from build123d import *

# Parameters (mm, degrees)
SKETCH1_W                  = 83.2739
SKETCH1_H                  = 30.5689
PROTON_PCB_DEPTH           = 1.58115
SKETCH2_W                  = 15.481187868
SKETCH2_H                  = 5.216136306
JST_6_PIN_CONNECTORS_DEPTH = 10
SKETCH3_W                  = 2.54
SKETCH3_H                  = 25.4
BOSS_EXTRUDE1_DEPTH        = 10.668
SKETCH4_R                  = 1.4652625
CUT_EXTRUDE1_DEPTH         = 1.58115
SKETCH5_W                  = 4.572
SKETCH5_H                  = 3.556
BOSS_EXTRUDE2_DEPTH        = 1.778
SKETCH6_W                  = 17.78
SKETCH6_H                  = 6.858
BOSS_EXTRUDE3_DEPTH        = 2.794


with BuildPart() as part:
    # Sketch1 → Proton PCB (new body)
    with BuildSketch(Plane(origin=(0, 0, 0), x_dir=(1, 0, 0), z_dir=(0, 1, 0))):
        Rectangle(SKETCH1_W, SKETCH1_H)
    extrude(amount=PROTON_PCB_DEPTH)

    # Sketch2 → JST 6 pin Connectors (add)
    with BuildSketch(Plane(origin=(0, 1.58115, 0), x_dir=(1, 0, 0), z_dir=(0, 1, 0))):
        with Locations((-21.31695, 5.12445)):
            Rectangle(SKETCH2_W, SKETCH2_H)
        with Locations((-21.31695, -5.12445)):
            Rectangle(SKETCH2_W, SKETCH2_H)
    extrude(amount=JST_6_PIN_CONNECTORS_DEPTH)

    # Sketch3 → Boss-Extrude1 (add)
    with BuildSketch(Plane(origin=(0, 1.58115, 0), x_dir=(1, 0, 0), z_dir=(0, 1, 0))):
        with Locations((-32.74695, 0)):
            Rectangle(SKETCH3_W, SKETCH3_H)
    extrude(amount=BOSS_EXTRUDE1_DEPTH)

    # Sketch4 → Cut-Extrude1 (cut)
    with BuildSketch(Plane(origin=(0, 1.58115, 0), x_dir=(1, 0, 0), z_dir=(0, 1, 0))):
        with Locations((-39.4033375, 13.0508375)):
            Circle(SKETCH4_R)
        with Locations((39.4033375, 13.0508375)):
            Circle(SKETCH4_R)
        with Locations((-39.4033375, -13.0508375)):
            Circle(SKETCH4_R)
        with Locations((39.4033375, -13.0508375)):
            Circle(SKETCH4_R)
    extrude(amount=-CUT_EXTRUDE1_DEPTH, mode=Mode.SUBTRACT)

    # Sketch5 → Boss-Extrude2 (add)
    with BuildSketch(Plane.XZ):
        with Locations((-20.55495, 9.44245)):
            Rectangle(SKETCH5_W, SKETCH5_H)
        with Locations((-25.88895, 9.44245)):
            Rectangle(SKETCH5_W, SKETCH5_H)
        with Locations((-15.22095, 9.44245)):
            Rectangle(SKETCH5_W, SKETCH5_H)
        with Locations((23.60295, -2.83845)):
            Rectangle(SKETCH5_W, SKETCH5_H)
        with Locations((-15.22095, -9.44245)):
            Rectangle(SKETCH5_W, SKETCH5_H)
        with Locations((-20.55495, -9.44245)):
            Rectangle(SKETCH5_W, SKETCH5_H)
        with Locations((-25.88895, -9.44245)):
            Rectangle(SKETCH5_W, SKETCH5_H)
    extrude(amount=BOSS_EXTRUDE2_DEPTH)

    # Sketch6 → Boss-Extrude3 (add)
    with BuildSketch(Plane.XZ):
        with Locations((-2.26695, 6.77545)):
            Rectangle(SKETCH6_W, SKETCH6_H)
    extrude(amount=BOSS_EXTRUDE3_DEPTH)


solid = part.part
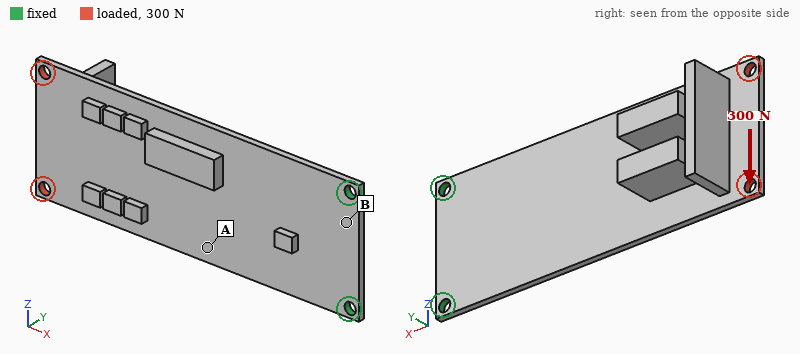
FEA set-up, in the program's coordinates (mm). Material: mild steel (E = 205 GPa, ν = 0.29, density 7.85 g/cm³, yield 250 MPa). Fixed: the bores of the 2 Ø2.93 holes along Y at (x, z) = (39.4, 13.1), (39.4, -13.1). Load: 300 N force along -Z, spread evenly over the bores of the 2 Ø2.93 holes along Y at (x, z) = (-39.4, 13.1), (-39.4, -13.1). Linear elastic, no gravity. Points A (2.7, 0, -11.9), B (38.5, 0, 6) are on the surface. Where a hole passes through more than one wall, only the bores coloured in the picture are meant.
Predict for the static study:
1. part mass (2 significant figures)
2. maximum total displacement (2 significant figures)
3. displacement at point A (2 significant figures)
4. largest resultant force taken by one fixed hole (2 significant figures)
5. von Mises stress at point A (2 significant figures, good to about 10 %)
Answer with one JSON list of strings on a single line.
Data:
["54 g", "78 µm", "24 µm", "920 N", "43 MPa"]
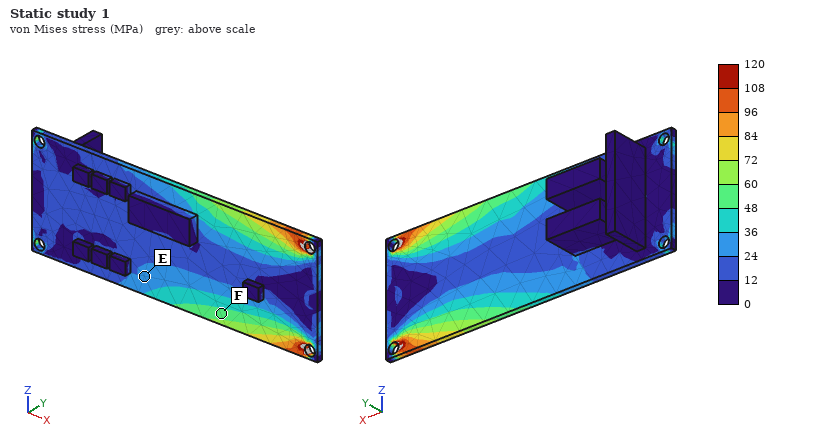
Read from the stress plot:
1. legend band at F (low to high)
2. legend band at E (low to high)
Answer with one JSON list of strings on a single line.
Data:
["48 to 60 MPa", "24 to 36 MPa"]
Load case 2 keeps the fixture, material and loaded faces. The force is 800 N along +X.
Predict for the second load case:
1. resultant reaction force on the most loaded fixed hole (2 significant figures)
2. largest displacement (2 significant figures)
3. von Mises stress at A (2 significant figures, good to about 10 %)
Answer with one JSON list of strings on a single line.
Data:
["420 N", "18 µm", "14 MPa"]
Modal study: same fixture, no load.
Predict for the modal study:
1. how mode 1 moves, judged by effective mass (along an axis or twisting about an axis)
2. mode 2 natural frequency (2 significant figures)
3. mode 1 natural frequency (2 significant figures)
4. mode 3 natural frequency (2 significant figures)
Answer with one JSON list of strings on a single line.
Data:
["along Y", "900 Hz", "130 Hz", "1300 Hz"]
